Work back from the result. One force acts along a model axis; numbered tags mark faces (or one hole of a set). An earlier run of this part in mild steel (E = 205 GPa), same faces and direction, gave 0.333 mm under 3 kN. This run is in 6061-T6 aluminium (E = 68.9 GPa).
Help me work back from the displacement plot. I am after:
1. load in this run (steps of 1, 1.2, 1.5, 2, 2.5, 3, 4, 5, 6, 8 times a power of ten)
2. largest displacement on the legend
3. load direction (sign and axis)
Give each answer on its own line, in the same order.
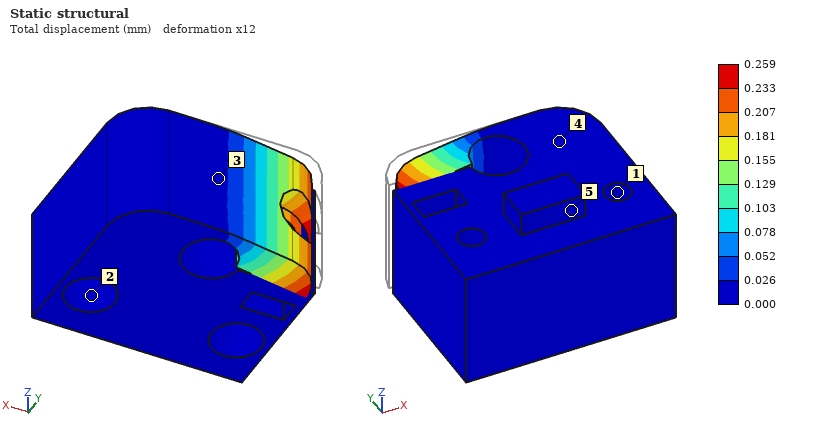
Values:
800 N
0.259 mm
-Y
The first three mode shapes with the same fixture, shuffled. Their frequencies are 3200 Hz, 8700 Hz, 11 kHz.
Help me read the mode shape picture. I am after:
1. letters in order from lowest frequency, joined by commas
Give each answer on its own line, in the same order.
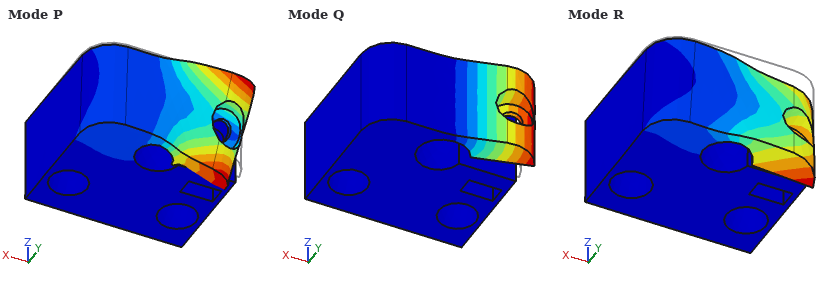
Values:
Q, R, P
